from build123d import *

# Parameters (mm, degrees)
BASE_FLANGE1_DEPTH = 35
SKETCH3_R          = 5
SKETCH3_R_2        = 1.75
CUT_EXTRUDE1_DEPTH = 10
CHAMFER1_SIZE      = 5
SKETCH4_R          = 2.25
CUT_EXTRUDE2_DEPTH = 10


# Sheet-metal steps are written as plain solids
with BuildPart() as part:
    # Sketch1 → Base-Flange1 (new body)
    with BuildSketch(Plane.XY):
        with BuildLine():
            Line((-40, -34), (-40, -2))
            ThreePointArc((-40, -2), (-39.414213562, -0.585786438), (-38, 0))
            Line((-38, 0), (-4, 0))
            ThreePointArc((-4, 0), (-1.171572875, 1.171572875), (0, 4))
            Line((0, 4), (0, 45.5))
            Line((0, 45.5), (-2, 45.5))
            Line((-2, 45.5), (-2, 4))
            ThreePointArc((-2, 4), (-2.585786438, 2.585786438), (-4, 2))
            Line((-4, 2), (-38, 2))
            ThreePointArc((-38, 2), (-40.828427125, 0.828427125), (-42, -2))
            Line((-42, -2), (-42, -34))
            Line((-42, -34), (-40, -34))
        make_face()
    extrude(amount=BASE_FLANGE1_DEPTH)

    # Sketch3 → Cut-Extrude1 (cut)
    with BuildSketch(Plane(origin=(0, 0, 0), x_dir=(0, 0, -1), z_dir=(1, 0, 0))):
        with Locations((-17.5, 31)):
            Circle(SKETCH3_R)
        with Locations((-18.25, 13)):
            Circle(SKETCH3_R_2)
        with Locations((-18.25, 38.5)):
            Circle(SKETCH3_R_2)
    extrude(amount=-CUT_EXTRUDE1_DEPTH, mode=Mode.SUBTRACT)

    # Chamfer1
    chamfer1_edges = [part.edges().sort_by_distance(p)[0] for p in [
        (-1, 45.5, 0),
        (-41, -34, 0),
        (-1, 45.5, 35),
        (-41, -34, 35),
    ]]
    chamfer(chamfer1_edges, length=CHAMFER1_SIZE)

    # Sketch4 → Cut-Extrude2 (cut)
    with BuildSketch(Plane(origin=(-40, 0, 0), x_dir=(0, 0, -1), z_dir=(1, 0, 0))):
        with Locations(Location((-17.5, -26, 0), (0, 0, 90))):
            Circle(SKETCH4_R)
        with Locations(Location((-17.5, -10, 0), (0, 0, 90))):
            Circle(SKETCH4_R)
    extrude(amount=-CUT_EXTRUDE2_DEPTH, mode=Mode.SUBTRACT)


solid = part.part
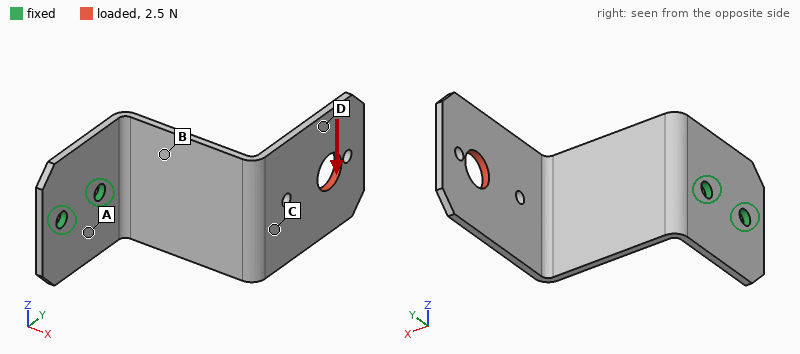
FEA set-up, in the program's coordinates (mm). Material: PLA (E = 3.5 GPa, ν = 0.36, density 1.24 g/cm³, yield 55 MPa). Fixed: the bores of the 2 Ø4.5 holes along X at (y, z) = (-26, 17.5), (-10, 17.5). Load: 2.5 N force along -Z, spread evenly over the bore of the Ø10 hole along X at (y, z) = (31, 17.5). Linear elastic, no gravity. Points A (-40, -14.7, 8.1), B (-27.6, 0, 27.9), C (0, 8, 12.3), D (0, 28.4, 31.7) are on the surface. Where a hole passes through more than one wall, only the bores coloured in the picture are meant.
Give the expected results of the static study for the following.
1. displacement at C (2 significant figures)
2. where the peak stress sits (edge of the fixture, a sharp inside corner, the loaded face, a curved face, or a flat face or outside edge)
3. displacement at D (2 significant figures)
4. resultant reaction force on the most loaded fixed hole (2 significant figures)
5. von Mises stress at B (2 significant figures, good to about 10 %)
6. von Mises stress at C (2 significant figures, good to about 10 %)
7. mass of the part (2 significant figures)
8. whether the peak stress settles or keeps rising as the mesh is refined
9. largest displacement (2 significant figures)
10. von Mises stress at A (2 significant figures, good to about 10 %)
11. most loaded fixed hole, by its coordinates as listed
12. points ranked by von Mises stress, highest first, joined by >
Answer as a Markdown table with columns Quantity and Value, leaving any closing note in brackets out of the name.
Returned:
| Quantity | Value |
|---|---|
| displacement at C | 0.33 mm |
| where the peak stress sits | edge of the fixture |
| displacement at D | 0.71 mm |
| resultant reaction force on the most loaded fixed hole | 7.2 N |
| von Mises stress at B | 2.1 MPa |
| von Mises stress at C | 0.76 MPa |
| mass of the part | 9.7 g |
| whether the peak stress settles or keeps rising as the mesh is refined | keeps rising |
| largest displacement | 0.98 mm |
| von Mises stress at A | 1.2 MPa |
| most loaded fixed hole, by its coordinates as listed | (-10, 17.5) |
| points ranked by von Mises stress, highest first, joined by > | B > A > C > D |
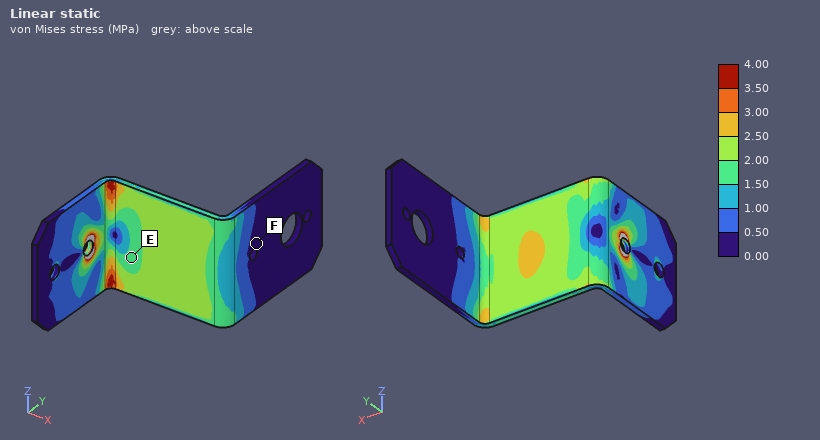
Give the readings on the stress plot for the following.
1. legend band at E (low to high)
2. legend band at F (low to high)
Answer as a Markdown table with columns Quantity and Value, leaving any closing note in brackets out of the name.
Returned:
| Quantity | Value |
|---|---|
| legend band at E | 1.50 to 2.00 MPa |
| legend band at F | 0.00 to 0.50 MPa |
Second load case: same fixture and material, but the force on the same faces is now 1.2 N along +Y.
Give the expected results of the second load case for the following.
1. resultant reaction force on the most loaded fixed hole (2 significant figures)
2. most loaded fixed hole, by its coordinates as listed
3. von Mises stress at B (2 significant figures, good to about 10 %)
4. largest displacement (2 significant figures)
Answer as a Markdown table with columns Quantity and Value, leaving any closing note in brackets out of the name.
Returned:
| Quantity | Value |
|---|---|
| resultant reaction force on the most loaded fixed hole | 1.5 N |
| most loaded fixed hole, by its coordinates as listed | (-10, 17.5) |
| von Mises stress at B | 1.3 MPa |
| largest displacement | 0.93 mm |
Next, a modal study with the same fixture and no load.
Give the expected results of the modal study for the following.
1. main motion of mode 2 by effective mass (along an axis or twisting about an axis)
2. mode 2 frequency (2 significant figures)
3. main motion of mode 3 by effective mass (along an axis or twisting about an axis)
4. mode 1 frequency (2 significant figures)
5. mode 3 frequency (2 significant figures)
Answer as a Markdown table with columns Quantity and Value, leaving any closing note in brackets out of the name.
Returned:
| Quantity | Value |
|---|---|
| main motion of mode 2 by effective mass | along Z |
| mode 2 frequency | 170 Hz |
| main motion of mode 3 by effective mass | along Y |
| mode 1 frequency | 89 Hz |
| mode 3 frequency | 280 Hz |
